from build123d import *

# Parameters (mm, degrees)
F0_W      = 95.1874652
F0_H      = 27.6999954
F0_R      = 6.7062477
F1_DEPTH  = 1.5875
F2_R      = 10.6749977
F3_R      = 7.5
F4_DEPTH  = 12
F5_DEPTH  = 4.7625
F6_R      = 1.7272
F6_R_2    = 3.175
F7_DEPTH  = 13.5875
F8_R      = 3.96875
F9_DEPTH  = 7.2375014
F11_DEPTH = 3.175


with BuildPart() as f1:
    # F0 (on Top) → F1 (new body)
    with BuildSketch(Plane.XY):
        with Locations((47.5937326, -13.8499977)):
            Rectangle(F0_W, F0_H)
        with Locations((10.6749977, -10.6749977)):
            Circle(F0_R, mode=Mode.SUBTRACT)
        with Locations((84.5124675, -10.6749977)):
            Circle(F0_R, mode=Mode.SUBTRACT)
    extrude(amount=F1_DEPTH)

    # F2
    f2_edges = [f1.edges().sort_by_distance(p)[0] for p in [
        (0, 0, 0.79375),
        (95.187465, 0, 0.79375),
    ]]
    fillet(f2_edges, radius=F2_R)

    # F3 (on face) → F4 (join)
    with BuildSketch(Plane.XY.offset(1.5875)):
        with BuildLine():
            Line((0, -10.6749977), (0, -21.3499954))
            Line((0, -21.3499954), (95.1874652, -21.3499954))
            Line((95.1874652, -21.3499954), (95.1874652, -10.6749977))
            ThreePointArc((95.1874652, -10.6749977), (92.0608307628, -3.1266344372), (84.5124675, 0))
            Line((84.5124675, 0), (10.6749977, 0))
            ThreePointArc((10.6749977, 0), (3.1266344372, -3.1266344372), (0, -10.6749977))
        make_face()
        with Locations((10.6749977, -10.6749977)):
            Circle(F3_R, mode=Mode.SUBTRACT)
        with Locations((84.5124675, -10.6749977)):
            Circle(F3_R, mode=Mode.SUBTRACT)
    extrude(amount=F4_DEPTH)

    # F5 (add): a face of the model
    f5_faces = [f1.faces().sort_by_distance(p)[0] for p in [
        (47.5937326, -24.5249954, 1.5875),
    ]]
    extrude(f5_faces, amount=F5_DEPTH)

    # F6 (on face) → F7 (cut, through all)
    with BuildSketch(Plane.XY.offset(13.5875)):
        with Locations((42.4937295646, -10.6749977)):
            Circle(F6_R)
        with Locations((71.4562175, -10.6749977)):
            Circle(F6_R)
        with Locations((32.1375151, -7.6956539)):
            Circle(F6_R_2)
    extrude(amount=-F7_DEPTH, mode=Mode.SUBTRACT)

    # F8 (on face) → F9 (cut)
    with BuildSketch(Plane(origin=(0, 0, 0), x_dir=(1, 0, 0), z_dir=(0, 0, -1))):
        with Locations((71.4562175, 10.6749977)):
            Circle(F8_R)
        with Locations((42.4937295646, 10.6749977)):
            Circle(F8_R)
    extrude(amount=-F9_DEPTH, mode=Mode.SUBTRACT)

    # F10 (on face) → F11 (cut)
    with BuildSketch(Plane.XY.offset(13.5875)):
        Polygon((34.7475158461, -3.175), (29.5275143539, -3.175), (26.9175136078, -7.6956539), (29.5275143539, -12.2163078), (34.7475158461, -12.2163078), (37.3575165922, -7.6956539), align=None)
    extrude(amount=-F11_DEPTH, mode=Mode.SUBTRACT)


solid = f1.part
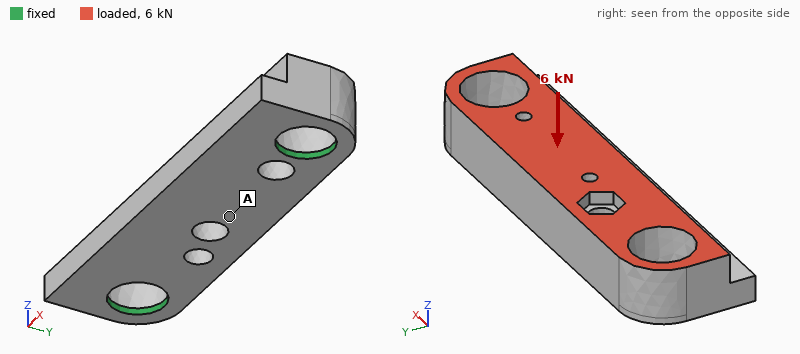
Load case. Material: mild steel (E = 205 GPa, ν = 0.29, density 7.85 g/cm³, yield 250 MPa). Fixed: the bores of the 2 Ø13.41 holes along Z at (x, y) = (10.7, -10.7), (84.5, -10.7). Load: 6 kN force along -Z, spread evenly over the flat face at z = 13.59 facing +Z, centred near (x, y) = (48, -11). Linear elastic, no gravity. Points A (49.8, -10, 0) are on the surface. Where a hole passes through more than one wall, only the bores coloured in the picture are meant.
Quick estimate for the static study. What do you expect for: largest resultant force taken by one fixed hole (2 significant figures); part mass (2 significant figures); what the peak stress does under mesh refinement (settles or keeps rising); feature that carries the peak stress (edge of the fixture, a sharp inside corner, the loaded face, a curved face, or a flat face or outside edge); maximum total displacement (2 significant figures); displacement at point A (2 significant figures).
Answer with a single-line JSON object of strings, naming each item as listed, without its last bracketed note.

{"largest resultant force taken by one fixed hole": "3.7 kN", "part mass": "190 g", "what the peak stress does under mesh refinement": "keeps rising", "feature that carries the peak stress": "edge of the fixture", "maximum total displacement": "13 µm", "displacement at point A": "12 µm"}
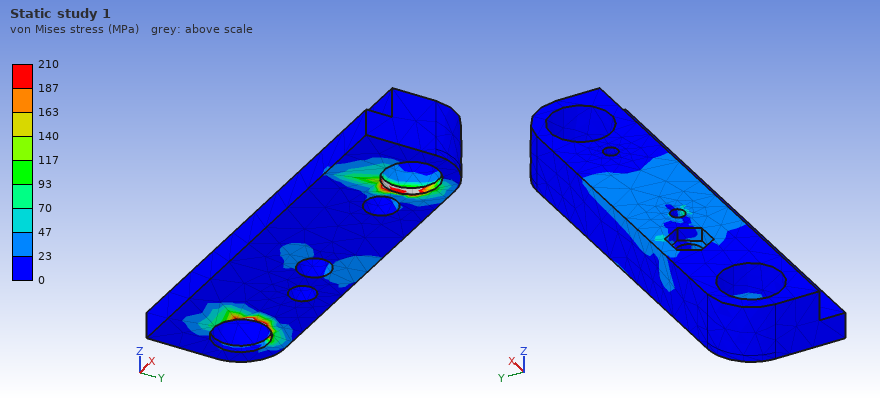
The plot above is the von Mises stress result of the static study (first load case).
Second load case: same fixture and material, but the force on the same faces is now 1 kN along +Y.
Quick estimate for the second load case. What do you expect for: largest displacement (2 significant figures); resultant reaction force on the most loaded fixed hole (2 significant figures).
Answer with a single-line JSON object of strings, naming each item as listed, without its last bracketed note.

{"largest displacement": "5.0 µm", "resultant reaction force on the most loaded fixed hole": "510 N"}
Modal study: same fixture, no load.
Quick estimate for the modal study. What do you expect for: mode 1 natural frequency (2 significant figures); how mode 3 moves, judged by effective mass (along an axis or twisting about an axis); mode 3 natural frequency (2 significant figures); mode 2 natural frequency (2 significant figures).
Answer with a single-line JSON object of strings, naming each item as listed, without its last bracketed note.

{"mode 1 natural frequency": "7800 Hz", "how mode 3 moves, judged by effective mass": "along Y", "mode 3 natural frequency": "13 kHz", "mode 2 natural frequency": "8900 Hz"}
